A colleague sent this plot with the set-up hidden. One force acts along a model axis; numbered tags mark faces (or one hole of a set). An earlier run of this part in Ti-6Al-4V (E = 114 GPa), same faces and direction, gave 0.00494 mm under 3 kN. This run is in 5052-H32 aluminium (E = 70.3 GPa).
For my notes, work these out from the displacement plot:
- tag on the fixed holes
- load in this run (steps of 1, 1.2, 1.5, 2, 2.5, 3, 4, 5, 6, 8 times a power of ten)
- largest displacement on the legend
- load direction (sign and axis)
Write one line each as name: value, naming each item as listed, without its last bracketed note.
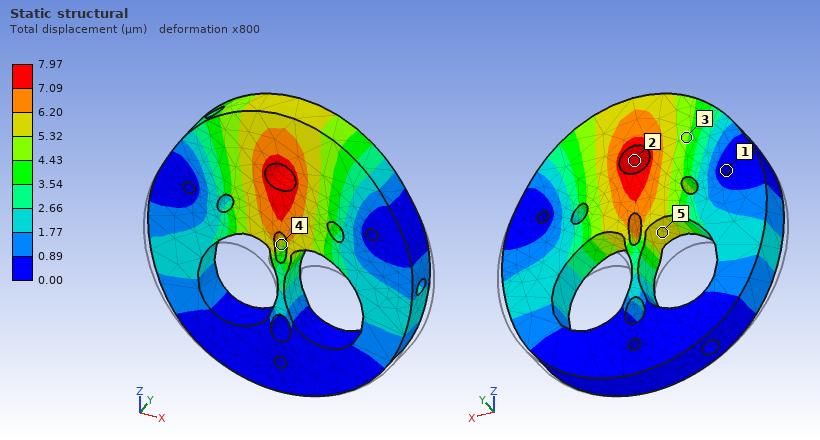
tag on the fixed holes: 1
load in this run: 3 kN
largest displacement on the legend: 7.97 µm
load direction: +Z
